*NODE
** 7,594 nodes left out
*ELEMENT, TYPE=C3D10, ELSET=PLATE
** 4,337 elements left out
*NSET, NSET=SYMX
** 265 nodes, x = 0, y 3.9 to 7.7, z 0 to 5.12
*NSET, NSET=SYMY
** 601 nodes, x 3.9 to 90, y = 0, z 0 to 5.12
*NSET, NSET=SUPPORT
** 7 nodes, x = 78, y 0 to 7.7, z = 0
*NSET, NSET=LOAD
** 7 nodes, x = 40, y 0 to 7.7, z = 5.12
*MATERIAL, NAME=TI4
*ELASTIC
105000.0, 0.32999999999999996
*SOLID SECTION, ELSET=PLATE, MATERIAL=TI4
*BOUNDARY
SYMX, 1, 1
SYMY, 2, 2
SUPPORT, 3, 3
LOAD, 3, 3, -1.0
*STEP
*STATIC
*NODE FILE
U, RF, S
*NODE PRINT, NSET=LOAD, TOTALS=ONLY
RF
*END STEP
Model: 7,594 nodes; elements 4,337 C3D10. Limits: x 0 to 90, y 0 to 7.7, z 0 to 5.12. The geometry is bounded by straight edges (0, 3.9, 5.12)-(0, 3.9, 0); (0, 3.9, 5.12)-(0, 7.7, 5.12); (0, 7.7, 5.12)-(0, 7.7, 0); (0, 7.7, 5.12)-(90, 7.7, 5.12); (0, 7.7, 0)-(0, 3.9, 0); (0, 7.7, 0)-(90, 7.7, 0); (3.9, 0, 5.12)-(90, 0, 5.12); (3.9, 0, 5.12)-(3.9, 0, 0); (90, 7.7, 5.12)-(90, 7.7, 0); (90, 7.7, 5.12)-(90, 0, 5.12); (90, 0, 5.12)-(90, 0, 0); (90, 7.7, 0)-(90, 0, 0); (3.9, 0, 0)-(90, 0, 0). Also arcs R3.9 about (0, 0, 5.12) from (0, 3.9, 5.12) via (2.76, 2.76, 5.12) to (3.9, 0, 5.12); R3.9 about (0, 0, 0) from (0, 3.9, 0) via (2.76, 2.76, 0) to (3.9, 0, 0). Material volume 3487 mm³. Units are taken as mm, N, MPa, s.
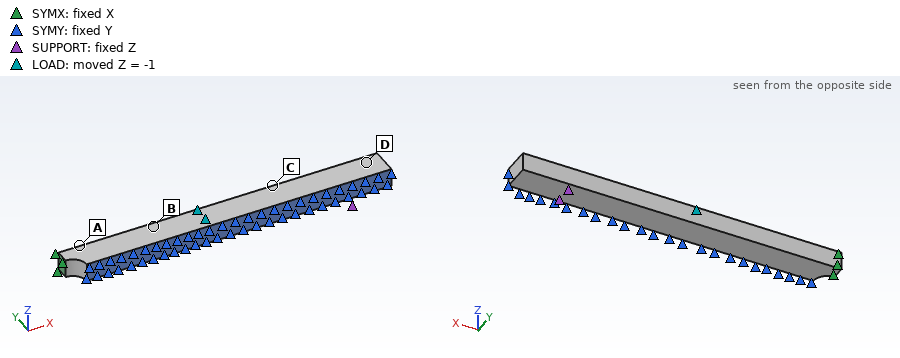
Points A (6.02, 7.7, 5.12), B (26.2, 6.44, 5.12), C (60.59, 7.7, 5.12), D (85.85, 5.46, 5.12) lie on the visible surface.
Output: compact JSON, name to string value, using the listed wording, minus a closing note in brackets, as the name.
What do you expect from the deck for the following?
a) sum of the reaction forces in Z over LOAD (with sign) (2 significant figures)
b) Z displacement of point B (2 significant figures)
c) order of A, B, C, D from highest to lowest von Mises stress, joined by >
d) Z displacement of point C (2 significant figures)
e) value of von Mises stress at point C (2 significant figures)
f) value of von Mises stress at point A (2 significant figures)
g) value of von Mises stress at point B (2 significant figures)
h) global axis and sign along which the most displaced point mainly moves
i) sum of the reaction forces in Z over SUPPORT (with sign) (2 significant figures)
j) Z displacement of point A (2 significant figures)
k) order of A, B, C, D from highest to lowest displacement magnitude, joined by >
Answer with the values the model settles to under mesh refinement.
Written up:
{"sum of the reaction forces in Z over LOAD (with sign)": "-110 N", "Z displacement of point B": "-1.2 mm", "order of A, B, C, D from highest to lowest von Mises stress, joined by >": "A > B > C > D", "Z displacement of point C": "-0.50 mm", "value of von Mises stress at point C": "57 MPa", "value of von Mises stress at point A": "160 MPa", "value of von Mises stress at point B": "120 MPa", "global axis and sign along which the most displaced point mainly moves": "-Z", "sum of the reaction forces in Z over SUPPORT (with sign)": "110 N", "Z displacement of point A": "-1.4 mm", "order of A, B, C, D from highest to lowest displacement magnitude, joined by >": "A > B > C > D"}
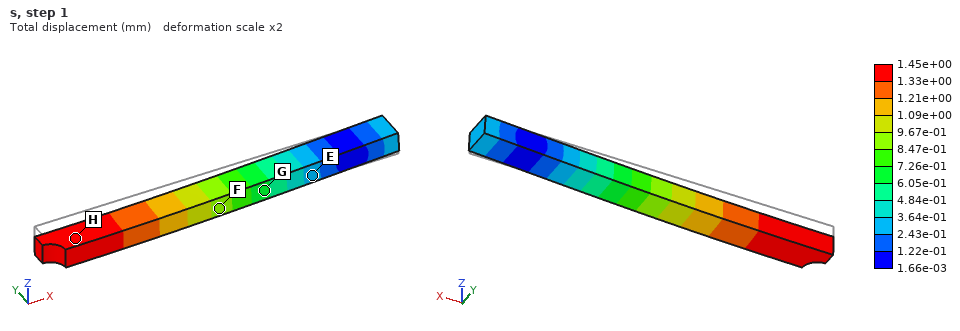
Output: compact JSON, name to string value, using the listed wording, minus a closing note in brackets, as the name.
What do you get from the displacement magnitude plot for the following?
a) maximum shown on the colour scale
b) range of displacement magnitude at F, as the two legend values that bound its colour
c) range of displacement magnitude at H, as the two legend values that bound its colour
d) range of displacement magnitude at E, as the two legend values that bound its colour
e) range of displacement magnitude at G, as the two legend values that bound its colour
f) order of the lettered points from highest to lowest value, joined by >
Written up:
{"maximum shown on the colour scale": "1.45e+00 mm", "range of displacement magnitude at F, as the two legend values that bound its colour": "8.47e-01 to 9.67e-01 mm", "range of displacement magnitude at H, as the two legend values that bound its colour": "1.33e+00 to 1.45e+00 mm", "range of displacement magnitude at E, as the two legend values that bound its colour": "2.43e-01 to 3.64e-01 mm", "range of displacement magnitude at G, as the two legend values that bound its colour": "6.05e-01 to 7.26e-01 mm", "order of the lettered points from highest to lowest value, joined by >": "H > F > G > E"}
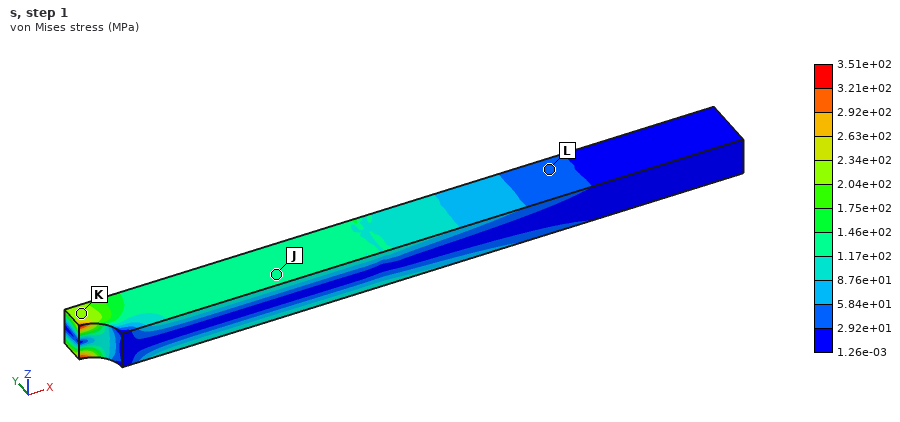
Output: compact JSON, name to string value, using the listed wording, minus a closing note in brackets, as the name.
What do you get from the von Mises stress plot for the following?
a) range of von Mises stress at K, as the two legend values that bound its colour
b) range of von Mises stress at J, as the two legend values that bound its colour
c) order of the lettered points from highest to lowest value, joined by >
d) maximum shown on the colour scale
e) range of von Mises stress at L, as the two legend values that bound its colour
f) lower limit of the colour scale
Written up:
{"range of von Mises stress at K, as the two legend values that bound its colour": "2.04e+02 to 2.34e+02 MPa", "range of von Mises stress at J, as the two legend values that bound its colour": "1.17e+02 to 1.46e+02 MPa", "order of the lettered points from highest to lowest value, joined by >": "K > J > L", "maximum shown on the colour scale": "3.51e+02 MPa", "range of von Mises stress at L, as the two legend values that bound its colour": "2.92e+01 to 5.84e+01 MPa", "lower limit of the colour scale": "1.26e-03 MPa"}
